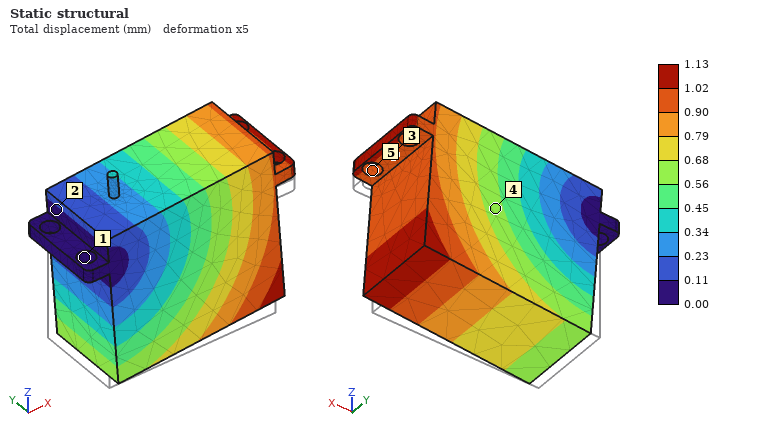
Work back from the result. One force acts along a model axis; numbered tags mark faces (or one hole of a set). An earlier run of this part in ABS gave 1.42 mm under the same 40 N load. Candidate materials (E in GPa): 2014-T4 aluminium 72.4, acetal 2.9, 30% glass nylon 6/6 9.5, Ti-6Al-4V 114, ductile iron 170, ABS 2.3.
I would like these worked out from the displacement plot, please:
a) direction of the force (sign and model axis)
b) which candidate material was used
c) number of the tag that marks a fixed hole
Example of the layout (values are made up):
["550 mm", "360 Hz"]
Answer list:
["+Z", "acetal", "1"]
